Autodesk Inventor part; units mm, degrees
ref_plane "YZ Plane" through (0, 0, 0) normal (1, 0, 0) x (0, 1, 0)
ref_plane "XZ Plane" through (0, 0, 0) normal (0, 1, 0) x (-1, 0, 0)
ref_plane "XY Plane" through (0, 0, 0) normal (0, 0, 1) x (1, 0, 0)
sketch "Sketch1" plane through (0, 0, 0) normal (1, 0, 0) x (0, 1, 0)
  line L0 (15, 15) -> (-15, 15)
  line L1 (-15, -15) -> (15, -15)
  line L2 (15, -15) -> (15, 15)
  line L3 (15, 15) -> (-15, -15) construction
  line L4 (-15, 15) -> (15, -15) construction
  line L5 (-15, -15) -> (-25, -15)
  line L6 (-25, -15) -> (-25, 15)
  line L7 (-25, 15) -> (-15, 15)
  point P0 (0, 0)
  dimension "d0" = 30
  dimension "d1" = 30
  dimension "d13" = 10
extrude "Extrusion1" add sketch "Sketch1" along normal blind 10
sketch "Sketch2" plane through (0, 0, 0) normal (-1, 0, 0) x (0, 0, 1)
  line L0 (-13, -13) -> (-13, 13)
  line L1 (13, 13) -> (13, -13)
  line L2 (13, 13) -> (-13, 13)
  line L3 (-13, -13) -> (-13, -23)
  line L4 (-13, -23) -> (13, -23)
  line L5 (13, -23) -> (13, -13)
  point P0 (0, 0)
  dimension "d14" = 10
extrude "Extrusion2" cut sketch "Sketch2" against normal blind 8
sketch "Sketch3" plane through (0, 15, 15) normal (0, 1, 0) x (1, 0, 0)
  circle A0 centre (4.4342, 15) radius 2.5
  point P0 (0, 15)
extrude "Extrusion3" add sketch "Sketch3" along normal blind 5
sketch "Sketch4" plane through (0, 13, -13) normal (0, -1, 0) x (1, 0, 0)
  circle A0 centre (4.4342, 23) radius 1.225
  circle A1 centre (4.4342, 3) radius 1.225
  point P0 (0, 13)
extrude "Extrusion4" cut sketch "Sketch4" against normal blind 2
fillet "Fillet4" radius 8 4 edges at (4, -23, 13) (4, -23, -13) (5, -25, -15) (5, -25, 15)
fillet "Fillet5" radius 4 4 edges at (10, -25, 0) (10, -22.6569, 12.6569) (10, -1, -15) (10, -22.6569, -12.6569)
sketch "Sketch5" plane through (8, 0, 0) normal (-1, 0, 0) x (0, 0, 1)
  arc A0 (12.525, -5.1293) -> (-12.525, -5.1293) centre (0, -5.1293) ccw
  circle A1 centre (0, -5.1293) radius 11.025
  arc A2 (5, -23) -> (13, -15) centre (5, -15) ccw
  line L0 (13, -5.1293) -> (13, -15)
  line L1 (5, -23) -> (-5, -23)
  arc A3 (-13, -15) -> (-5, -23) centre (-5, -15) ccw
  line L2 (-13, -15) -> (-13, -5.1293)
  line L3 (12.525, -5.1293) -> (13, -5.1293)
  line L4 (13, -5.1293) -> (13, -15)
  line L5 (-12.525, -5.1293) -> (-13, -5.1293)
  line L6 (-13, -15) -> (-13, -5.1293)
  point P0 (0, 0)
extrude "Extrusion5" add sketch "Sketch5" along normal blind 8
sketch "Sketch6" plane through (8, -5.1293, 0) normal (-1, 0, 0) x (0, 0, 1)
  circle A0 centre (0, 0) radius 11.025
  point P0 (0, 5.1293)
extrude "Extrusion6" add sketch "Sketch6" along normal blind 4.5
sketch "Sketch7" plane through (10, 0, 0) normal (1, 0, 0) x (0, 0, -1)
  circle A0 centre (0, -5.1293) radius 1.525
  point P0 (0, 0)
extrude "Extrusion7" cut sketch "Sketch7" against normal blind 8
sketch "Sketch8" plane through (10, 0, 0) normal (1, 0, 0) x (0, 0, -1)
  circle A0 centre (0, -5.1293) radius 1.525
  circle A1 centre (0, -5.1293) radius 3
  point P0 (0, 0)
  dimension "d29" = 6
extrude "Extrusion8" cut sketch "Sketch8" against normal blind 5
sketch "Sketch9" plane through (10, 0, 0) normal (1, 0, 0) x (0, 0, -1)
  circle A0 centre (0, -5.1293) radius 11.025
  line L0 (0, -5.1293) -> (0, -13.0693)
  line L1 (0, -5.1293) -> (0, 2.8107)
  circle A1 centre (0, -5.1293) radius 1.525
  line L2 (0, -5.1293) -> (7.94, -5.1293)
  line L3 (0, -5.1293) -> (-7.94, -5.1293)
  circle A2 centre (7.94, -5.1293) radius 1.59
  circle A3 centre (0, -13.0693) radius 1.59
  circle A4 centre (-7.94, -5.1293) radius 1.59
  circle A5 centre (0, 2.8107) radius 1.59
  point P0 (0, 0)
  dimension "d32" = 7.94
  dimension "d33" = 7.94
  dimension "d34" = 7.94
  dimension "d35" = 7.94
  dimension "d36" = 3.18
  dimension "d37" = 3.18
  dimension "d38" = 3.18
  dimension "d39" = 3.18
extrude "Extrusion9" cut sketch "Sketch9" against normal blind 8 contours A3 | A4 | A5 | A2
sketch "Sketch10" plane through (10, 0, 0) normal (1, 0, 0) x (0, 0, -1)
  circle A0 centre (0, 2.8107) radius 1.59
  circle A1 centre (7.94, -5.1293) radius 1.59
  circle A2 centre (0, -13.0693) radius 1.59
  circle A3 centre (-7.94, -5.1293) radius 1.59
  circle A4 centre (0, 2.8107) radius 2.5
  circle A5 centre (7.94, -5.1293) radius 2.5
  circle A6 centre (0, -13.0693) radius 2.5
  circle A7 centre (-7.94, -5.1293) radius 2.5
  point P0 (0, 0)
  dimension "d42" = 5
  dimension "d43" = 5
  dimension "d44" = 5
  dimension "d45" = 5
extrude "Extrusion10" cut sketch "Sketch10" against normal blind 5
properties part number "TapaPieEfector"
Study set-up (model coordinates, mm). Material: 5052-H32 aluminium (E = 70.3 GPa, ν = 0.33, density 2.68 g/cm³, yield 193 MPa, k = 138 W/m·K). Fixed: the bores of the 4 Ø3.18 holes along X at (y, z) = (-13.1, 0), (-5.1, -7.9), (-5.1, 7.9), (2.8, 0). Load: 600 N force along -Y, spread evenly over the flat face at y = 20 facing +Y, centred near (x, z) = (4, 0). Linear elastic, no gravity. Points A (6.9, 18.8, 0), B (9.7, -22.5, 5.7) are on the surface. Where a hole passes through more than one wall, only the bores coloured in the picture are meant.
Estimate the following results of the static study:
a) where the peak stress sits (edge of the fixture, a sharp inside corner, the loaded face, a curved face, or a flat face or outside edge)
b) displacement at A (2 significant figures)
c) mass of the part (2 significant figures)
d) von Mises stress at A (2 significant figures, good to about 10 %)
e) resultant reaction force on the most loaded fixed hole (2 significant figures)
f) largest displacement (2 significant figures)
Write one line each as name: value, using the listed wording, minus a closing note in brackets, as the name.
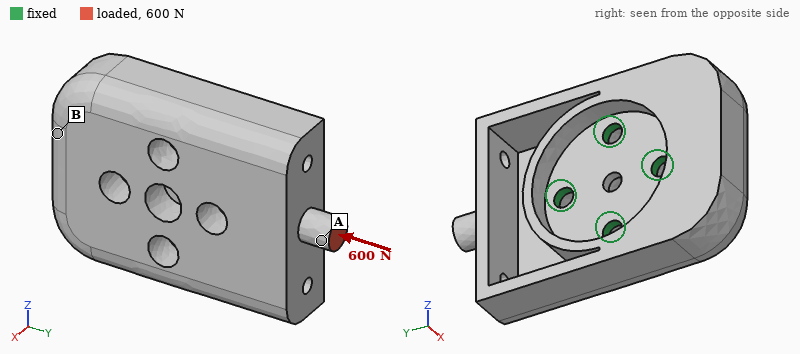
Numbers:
where the peak stress sits: a curved face
displacement at A: 0.073 mm
mass of the part: 21 g
von Mises stress at A: 29 MPa
resultant reaction force on the most loaded fixed hole: 200 N
largest displacement: 0.11 mm
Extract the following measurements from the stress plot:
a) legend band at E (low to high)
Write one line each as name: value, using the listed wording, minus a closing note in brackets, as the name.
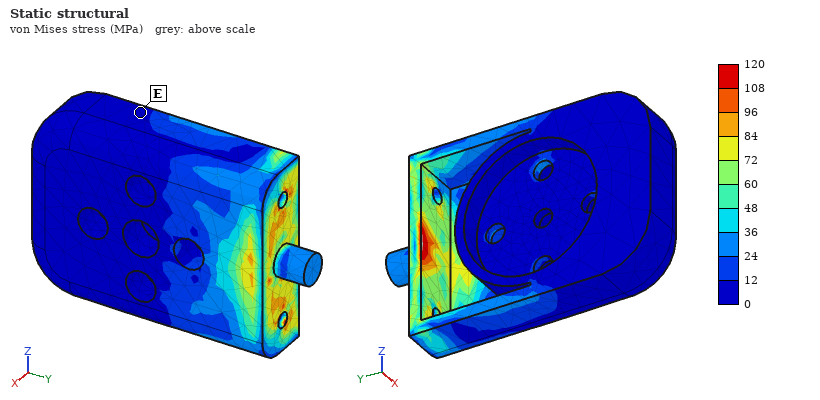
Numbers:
legend band at E: 0 to 12 MPa
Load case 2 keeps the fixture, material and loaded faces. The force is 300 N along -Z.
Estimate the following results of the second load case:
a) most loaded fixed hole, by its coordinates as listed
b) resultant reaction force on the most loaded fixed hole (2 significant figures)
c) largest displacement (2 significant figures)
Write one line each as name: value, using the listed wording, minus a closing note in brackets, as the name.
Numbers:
most loaded fixed hole, by its coordinates as listed: (2.8, 0)
resultant reaction force on the most loaded fixed hole: 340 N
largest displacement: 40 µm
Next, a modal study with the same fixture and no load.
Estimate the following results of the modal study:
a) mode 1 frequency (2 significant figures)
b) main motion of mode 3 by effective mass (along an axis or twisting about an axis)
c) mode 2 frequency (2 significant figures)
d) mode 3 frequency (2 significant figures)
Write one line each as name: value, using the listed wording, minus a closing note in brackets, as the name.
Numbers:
mode 1 frequency: 9600 Hz
main motion of mode 3 by effective mass: along X
mode 2 frequency: 12 kHz
mode 3 frequency: 14 kHz
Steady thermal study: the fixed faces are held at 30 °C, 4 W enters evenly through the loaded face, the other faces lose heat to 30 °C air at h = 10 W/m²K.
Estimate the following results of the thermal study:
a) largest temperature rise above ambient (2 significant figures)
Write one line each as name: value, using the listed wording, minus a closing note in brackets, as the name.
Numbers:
largest temperature rise above ambient: 17 K
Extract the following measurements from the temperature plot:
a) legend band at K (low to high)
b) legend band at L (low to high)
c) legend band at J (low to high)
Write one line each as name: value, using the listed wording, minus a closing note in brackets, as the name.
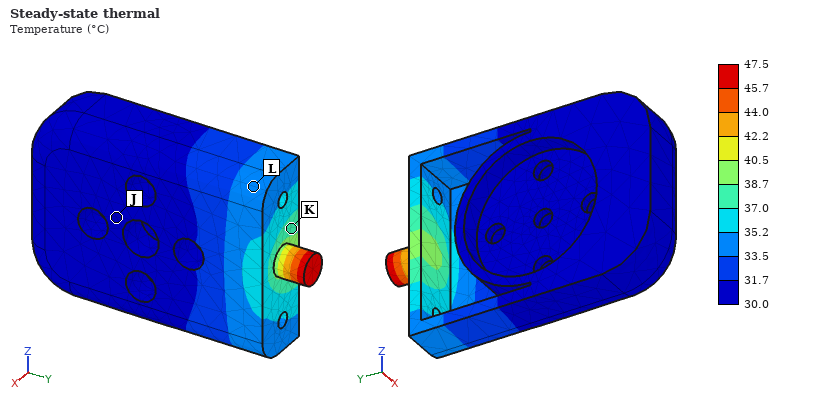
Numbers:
legend band at K: 37.0 to 38.7 °C
legend band at L: 33.5 to 35.2 °C
legend band at J: 30.0 to 31.7 °C
